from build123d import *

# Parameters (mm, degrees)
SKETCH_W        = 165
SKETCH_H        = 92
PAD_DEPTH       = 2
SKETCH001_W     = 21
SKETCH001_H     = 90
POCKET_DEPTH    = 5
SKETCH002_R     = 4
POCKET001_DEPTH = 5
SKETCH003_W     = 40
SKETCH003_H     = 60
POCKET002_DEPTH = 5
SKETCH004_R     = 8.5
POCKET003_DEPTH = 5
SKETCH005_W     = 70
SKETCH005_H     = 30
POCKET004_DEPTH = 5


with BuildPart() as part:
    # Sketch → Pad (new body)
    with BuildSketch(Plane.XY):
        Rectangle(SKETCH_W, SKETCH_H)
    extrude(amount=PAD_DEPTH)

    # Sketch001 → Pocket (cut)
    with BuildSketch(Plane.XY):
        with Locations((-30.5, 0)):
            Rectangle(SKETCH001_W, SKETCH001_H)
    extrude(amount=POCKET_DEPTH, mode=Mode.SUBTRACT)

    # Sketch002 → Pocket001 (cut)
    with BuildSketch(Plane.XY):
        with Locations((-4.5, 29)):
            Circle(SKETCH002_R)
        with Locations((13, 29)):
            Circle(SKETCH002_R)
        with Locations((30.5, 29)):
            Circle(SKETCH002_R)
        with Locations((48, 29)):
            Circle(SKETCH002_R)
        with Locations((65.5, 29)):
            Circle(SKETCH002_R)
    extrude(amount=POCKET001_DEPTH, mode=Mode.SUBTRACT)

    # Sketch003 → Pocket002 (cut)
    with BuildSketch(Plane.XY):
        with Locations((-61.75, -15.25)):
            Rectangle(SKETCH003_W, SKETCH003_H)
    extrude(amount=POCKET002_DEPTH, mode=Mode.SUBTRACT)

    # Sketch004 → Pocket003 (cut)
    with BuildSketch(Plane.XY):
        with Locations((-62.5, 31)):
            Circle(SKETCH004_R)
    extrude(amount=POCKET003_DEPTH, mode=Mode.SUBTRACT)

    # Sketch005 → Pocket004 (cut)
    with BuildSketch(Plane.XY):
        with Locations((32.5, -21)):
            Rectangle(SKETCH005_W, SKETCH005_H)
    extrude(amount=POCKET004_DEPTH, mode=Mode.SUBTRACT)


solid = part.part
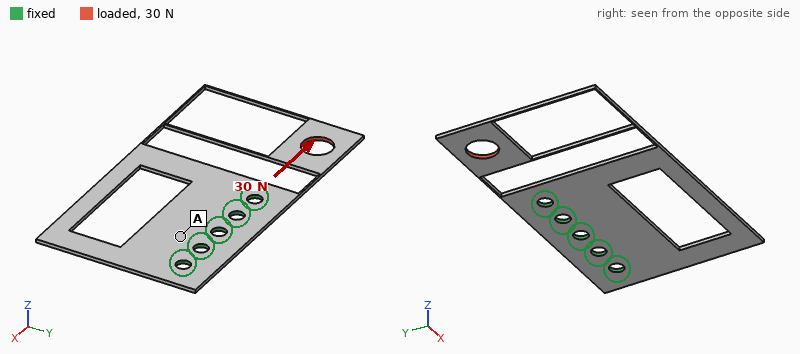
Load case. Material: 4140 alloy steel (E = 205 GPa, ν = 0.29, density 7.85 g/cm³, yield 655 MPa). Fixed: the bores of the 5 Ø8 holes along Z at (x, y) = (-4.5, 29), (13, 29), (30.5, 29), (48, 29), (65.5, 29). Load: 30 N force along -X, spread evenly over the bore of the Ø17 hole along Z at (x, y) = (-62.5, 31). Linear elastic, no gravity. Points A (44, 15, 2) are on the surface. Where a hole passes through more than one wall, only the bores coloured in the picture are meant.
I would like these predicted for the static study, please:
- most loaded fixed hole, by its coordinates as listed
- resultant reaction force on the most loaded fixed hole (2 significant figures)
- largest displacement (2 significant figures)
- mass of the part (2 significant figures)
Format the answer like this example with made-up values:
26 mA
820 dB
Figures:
(-4.5, 29)
15 N
2.0 mm
130 g
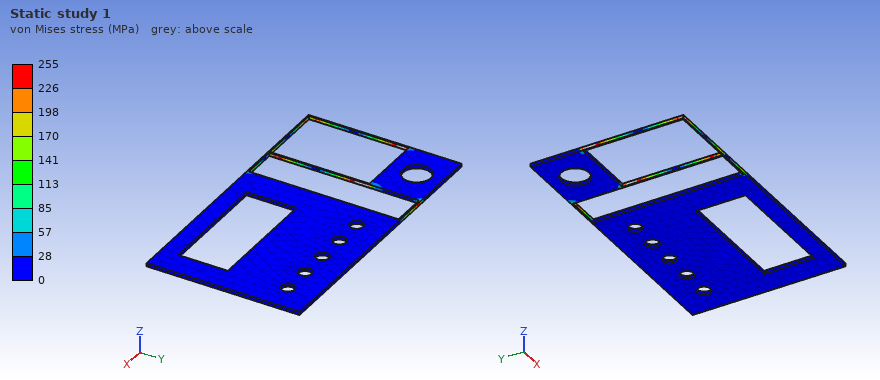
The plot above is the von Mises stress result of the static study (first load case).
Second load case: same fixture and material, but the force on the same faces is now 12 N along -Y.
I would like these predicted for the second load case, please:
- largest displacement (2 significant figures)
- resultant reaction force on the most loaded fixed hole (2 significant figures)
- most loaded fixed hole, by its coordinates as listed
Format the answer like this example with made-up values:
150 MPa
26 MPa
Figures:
1.8 mm
21 N
(-4.5, 29)
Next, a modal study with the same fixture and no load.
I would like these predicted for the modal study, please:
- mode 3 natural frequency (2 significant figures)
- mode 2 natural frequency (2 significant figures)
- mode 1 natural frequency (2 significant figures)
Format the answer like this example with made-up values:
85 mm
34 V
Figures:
280 Hz
110 Hz
93 Hz
